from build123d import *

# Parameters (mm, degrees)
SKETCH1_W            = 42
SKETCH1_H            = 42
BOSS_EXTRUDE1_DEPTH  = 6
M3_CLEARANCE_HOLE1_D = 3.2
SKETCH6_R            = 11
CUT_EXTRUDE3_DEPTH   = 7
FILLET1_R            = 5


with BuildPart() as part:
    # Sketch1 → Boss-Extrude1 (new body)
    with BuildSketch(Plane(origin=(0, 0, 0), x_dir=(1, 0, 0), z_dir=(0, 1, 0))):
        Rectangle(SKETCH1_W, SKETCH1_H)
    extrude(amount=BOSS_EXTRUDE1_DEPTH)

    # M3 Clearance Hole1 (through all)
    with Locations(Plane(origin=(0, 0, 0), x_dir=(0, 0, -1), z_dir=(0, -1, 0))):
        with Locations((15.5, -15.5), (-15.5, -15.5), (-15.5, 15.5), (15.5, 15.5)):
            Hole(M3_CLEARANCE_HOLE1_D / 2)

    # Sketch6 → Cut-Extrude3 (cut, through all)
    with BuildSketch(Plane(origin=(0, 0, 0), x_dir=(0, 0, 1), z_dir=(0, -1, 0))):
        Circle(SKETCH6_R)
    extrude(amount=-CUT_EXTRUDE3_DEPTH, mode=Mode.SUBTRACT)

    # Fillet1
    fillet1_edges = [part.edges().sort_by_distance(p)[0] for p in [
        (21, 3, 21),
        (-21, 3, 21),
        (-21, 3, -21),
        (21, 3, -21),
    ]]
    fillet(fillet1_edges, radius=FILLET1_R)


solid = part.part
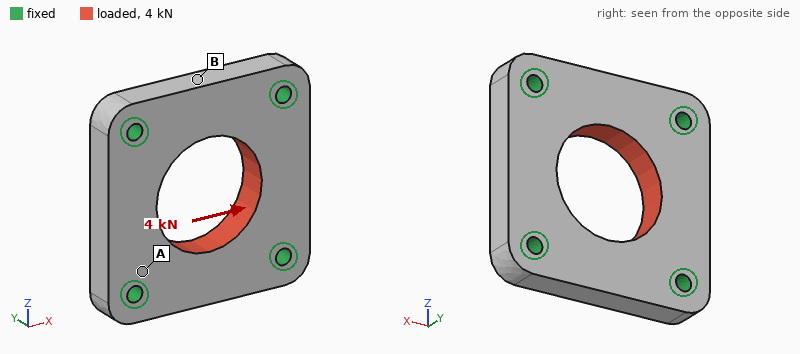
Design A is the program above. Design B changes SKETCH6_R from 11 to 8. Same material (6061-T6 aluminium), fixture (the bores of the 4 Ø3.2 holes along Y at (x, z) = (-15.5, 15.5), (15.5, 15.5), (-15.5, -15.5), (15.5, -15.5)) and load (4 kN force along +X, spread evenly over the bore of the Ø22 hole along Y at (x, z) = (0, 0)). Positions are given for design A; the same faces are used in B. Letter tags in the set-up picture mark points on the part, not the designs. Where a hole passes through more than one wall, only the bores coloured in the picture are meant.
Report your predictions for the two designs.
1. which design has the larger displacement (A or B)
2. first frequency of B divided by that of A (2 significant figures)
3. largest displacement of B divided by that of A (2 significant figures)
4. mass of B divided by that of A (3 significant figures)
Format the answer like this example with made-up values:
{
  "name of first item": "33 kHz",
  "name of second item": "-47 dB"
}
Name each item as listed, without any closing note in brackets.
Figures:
{
  "which design has the larger displacement": "A",
  "first frequency of B divided by that of A": "0.84",
  "largest displacement of B divided by that of A": "0.90",
  "mass of B divided by that of A": "1.13"
}
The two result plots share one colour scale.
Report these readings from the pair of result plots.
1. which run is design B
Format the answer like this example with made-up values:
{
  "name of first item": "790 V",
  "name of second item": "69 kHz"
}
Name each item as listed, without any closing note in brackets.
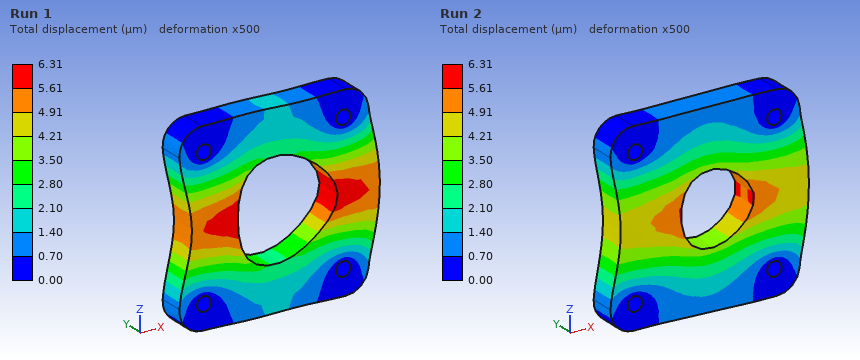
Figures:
{
  "which run is design B": "Run 2"
}
